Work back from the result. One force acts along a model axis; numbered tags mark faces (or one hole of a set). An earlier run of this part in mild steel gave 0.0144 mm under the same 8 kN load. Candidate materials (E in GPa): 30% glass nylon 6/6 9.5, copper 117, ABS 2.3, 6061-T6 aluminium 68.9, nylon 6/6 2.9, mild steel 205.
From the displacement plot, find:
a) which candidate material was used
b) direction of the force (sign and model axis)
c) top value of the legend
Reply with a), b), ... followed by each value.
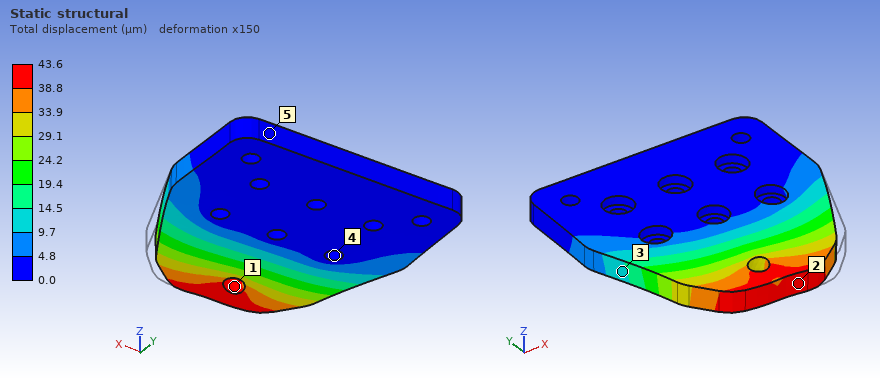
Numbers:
a) 6061-T6 aluminium
b) -X
c) 43.6 µm
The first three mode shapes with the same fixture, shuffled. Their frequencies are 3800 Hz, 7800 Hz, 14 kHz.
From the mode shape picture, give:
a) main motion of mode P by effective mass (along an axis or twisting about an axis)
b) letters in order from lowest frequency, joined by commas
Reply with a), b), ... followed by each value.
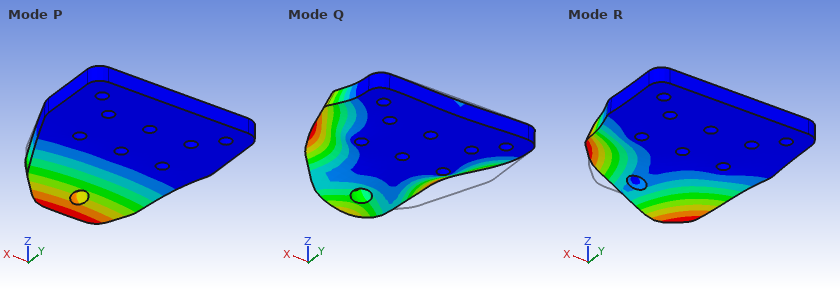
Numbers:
a) along Z
b) P, R, Q
